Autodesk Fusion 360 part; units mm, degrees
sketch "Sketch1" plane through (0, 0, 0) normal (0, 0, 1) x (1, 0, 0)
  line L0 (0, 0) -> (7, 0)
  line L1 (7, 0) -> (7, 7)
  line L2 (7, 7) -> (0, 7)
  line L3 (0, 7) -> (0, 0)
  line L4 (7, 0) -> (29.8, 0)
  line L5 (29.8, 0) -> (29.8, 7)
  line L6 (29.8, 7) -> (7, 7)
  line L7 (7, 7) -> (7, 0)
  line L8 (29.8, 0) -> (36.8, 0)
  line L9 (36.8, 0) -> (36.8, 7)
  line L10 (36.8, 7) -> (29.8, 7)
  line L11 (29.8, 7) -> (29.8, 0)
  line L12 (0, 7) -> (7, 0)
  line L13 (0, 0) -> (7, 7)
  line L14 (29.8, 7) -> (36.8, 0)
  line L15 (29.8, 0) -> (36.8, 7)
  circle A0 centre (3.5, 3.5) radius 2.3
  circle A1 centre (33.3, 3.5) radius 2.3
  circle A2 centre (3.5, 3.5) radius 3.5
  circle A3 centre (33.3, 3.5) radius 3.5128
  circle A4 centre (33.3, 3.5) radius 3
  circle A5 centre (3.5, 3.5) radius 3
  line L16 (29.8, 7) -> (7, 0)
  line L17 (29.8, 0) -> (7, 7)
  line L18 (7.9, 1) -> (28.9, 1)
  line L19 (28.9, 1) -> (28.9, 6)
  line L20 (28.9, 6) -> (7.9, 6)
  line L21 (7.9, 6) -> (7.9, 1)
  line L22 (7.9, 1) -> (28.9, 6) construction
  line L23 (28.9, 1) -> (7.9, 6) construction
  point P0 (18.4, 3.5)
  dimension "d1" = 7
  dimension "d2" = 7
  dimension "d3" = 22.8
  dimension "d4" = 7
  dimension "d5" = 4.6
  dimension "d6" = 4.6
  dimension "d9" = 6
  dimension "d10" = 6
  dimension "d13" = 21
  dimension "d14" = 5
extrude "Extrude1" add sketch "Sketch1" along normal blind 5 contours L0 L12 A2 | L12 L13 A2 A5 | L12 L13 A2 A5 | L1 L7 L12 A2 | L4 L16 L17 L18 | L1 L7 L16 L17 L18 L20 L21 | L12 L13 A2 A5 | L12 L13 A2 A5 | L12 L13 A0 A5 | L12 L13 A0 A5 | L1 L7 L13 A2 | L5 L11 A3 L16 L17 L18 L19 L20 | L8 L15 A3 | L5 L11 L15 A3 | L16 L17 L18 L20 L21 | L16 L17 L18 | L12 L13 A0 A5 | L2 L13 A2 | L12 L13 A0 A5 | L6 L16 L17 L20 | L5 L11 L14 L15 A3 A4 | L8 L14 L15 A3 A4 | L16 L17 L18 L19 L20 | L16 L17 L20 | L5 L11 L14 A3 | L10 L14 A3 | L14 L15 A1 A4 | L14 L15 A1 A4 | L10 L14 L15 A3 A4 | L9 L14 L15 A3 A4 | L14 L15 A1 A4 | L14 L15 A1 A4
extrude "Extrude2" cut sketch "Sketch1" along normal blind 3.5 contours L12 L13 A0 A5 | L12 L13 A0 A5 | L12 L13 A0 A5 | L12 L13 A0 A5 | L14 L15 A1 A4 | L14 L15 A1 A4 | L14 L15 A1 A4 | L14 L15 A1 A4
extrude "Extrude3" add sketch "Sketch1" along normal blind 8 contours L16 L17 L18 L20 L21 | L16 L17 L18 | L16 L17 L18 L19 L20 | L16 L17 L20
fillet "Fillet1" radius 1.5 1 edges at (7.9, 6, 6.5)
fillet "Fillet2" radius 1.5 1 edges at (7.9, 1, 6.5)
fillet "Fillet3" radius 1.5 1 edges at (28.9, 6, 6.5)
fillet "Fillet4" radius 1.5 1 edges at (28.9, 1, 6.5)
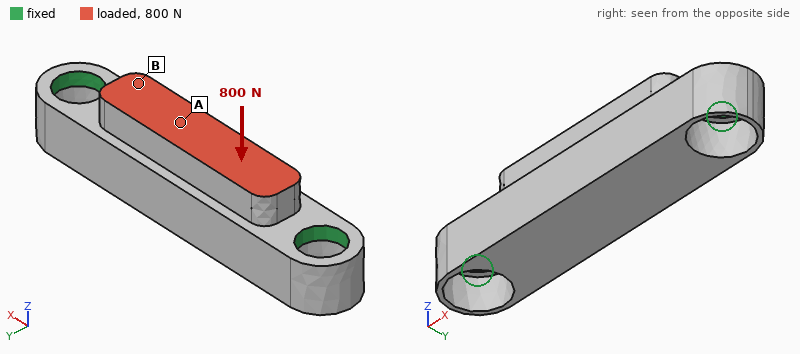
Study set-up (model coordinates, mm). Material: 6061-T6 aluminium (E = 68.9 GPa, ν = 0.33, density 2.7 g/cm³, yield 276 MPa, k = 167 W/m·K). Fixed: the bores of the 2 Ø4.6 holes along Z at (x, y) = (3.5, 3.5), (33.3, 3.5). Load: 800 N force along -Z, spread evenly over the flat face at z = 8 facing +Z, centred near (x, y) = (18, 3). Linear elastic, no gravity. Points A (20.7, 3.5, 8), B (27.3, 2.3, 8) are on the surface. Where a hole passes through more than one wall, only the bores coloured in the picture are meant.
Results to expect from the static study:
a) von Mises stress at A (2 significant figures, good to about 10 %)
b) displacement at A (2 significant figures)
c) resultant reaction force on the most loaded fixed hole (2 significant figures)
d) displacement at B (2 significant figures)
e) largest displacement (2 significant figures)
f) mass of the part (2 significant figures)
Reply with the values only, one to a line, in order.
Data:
36 MPa
14 µm
420 N
9.5 µm
15 µm
3.5 g
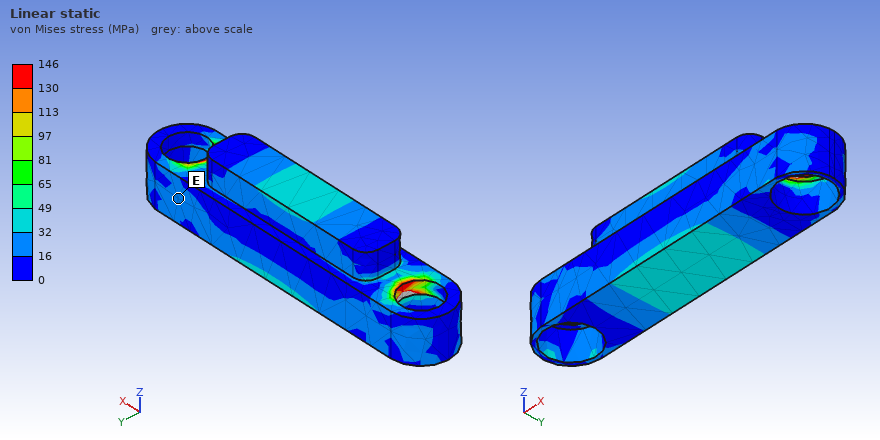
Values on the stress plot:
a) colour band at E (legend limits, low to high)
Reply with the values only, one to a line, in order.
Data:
16 to 32 MPa
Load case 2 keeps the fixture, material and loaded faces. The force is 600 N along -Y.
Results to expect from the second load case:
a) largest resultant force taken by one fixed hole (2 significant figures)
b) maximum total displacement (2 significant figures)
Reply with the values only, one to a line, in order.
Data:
300 N
31 µm
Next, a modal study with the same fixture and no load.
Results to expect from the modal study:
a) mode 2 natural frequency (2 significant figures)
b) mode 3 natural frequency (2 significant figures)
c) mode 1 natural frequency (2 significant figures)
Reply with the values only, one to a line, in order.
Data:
24 kHz
27 kHz
23 kHz
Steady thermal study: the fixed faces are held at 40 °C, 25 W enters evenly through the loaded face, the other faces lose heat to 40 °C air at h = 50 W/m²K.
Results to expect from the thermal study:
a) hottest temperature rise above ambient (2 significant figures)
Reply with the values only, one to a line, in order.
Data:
26 K
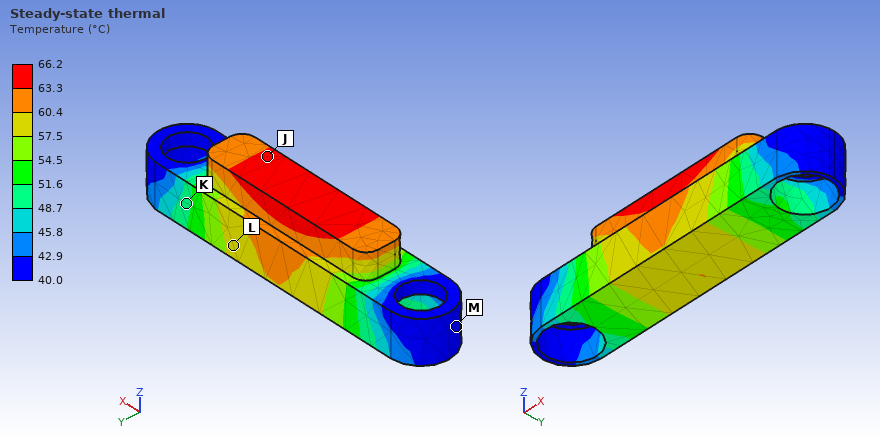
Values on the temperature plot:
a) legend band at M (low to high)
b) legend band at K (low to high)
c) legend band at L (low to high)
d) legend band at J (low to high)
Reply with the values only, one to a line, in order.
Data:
40.0 to 42.9 °C
48.7 to 51.6 °C
57.5 to 60.4 °C
63.3 to 66.2 °C
